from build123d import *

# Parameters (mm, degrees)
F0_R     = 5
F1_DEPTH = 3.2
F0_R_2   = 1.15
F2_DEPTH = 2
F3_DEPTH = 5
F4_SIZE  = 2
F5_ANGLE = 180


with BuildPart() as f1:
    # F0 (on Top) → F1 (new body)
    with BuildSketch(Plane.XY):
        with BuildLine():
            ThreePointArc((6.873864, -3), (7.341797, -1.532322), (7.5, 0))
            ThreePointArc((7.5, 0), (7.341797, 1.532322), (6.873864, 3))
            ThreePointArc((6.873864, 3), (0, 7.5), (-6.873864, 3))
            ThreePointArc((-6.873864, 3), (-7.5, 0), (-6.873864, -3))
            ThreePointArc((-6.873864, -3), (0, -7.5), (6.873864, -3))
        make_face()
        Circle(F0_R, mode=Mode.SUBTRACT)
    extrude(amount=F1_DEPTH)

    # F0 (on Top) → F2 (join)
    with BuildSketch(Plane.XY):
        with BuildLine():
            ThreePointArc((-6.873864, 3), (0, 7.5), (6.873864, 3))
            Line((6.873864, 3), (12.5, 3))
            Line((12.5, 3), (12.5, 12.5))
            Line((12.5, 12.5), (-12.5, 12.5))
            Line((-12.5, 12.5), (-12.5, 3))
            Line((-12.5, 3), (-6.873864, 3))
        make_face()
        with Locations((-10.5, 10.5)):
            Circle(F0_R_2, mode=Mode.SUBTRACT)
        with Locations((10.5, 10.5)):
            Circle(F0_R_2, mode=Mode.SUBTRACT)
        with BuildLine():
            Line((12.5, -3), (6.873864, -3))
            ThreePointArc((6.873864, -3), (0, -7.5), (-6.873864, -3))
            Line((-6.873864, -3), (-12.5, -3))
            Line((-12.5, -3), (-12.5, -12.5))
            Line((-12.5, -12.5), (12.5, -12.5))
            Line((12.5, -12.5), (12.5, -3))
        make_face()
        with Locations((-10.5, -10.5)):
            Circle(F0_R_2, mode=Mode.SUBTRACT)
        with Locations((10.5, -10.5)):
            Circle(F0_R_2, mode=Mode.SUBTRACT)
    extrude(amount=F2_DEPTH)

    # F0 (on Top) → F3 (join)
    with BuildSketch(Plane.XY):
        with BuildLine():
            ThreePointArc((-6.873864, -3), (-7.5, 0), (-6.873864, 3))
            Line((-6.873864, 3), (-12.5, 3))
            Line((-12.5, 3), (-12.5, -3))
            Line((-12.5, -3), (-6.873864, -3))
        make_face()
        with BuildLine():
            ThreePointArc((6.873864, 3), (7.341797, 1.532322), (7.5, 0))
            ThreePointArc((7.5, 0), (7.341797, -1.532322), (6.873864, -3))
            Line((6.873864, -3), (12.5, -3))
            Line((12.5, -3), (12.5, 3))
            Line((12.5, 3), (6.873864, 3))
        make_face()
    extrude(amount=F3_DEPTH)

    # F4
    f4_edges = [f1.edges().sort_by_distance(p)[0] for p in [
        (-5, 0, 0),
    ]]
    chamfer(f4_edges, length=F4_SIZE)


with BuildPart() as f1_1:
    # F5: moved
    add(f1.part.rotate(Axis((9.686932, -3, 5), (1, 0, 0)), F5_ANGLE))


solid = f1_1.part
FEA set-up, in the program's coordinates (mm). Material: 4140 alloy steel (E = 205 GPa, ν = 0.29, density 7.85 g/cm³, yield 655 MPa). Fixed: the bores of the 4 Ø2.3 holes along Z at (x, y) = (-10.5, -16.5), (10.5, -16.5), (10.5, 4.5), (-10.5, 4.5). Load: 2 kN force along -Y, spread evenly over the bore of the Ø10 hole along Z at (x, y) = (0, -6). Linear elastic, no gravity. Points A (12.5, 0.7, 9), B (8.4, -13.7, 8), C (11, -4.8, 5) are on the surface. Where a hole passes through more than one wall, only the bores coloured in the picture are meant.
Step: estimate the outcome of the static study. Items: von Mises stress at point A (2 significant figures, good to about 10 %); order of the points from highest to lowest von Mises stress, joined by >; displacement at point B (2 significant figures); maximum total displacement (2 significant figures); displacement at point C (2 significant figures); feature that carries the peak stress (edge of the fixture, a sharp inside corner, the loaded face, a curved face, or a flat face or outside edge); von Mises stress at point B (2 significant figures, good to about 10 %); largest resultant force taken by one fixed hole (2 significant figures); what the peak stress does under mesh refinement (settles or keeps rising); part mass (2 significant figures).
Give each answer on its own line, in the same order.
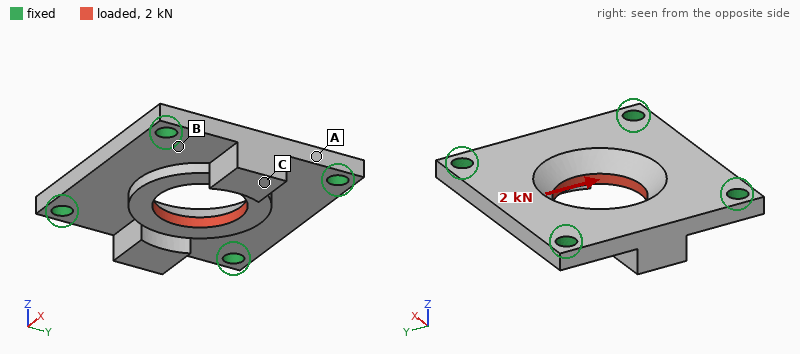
32 MPa
B > A > C
1.0 µm
5.6 µm
2.0 µm
edge of the fixture
59 MPa
550 N
keeps rising
10 g
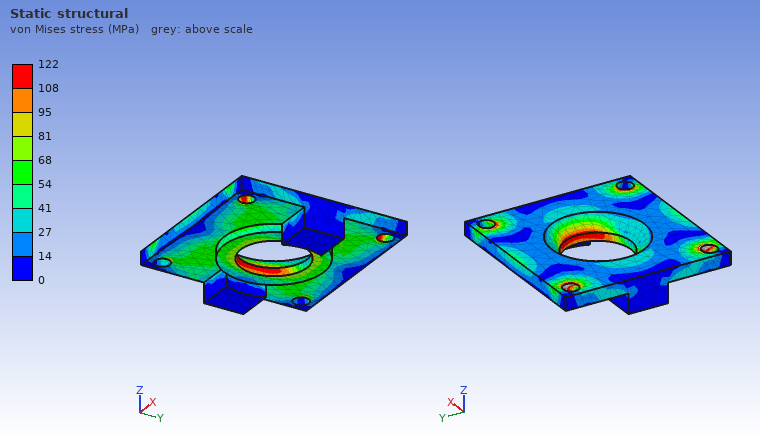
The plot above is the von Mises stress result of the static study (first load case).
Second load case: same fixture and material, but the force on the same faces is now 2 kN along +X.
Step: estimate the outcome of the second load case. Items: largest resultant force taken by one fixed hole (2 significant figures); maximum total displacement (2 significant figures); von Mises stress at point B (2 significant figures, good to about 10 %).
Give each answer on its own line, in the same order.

550 N
6.0 µm
59 MPa
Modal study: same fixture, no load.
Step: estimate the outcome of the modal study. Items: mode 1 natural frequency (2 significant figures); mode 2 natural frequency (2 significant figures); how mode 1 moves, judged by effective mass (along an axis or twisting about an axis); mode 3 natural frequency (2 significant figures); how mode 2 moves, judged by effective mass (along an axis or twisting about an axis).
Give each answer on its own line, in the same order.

19 kHz
23 kHz
along Z
26 kHz
twisting about Y
